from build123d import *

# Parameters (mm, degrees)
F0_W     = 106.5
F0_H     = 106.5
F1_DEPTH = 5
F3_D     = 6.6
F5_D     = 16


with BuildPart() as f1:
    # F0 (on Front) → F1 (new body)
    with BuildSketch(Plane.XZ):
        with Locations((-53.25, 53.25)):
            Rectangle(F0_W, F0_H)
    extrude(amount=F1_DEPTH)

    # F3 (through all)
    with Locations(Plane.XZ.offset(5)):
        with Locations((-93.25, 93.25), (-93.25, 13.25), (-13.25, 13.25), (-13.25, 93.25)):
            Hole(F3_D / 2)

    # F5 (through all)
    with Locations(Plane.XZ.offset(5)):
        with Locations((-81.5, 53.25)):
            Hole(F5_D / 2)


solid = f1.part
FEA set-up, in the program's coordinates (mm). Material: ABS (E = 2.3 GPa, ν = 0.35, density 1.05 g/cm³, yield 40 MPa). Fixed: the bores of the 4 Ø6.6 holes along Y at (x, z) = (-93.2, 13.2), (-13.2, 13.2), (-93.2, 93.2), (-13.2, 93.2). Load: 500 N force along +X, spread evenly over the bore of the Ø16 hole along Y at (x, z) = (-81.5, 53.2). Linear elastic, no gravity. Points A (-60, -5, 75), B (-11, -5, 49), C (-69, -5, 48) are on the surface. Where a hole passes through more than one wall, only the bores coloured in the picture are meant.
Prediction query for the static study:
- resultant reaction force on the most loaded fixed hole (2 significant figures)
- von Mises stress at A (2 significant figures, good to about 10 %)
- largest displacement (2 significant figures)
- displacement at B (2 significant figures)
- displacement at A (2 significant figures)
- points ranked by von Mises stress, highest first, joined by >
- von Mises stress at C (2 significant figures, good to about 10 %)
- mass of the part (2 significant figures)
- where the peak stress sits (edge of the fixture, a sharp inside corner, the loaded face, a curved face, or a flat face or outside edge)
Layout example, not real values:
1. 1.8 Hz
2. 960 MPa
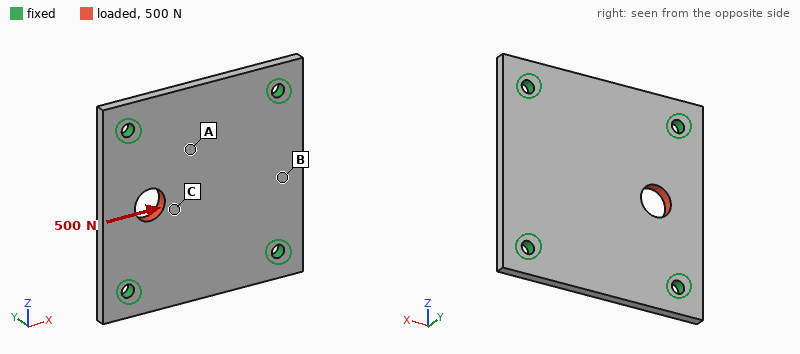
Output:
1. 150 N
2. 1.2 MPa
3. 55 µm
4. 14 µm
5. 19 µm
6. C > A > B
7. 2.0 MPa
8. 58 g
9. edge of the fixture
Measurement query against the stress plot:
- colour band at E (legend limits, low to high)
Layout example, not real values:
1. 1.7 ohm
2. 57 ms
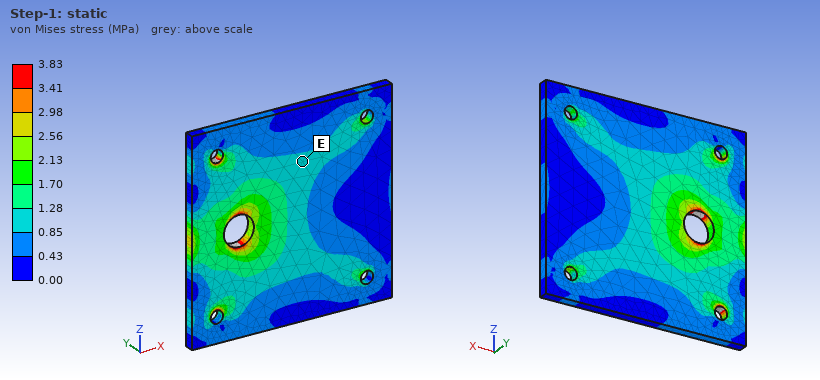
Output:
1. 0.85 to 1.28 MPa
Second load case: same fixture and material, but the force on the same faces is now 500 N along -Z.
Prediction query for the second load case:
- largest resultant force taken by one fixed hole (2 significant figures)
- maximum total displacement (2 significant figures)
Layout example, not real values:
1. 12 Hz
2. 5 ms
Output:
1. 200 N
2. 31 µm
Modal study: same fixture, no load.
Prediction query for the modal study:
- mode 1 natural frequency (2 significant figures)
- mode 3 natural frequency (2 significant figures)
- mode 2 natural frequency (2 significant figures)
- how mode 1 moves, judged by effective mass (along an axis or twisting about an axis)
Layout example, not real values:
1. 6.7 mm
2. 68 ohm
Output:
1. 850 Hz
2. 1300 Hz
3. 1300 Hz
4. along Y
